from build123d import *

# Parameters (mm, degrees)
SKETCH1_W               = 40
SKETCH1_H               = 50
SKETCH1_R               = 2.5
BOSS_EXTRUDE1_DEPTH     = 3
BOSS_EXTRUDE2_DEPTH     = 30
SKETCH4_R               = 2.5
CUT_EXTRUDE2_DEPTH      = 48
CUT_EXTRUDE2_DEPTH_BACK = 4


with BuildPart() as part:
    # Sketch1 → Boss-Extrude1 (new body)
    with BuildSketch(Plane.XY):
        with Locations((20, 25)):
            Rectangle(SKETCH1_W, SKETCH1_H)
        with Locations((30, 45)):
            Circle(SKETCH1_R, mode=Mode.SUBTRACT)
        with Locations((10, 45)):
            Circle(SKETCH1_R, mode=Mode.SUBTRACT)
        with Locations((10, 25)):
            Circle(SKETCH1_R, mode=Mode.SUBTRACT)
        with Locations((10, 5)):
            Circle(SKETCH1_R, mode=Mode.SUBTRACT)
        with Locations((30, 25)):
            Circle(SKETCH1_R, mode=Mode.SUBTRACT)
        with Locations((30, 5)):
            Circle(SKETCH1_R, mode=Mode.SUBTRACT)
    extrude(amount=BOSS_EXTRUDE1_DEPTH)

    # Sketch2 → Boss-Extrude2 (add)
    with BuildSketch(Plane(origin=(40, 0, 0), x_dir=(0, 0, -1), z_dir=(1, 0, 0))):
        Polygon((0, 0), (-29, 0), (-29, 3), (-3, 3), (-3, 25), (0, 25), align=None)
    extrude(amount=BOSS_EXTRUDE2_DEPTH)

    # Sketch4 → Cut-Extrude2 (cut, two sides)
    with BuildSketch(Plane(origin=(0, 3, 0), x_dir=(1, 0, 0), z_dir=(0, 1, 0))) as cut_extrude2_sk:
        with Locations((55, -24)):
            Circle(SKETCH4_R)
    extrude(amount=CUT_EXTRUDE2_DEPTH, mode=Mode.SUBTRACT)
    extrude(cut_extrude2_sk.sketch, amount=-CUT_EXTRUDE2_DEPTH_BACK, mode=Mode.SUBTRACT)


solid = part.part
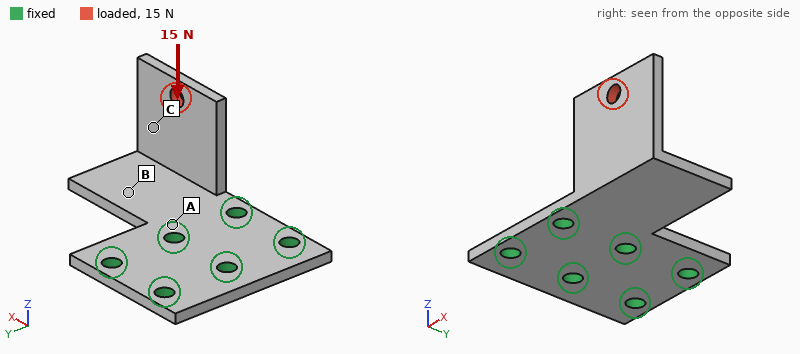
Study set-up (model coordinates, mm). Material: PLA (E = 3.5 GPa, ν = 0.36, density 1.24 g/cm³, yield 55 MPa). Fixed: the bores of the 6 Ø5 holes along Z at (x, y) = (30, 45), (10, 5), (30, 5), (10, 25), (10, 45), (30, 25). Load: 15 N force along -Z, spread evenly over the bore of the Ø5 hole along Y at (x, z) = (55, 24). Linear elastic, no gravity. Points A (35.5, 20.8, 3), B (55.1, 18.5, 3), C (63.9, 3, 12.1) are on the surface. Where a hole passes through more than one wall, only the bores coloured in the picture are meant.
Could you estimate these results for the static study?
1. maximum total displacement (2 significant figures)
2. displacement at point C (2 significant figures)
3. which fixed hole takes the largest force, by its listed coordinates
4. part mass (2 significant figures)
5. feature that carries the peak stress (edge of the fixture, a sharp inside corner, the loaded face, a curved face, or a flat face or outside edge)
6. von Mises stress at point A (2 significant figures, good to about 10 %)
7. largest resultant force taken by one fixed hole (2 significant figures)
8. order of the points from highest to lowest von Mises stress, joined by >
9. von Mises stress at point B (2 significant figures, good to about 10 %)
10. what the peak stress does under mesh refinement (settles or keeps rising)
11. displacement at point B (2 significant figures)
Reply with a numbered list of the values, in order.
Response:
1. 0.89 mm
2. 0.59 mm
3. (30, 5)
4. 13 g
5. edge of the fixture
6. 4.6 MPa
7. 18 N
8. A > B > C
9. 1.8 MPa
10. keeps rising
11. 0.25 mm
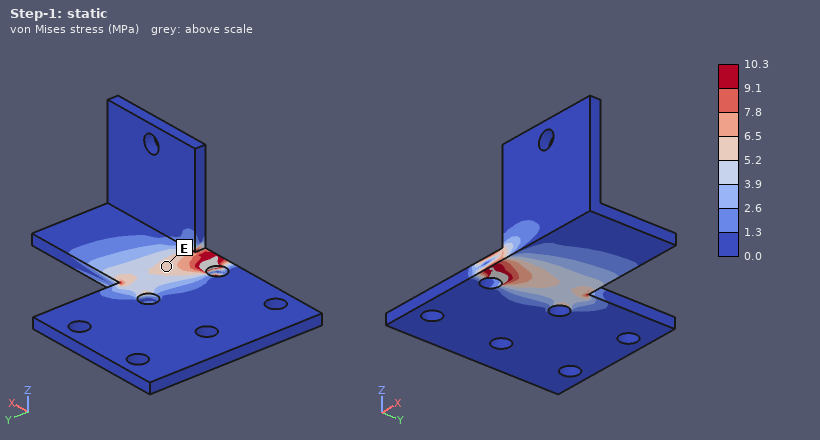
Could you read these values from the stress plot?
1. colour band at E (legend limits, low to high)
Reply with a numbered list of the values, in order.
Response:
1. 5.2 to 6.5 MPa
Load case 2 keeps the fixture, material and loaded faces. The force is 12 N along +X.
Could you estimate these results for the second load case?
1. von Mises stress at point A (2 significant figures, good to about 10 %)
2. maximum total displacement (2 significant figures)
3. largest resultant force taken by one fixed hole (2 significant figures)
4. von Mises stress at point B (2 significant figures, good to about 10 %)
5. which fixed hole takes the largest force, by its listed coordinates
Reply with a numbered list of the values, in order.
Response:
1. 4.4 MPa
2. 0.89 mm
3. 13 N
4. 1.9 MPa
5. (30, 5)
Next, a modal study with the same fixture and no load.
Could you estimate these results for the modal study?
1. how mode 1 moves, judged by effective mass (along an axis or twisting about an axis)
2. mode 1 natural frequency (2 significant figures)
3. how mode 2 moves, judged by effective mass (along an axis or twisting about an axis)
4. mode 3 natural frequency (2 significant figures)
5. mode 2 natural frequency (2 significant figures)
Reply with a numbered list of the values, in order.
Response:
1. along Z
2. 350 Hz
3. along Y
4. 1800 Hz
5. 640 Hz
